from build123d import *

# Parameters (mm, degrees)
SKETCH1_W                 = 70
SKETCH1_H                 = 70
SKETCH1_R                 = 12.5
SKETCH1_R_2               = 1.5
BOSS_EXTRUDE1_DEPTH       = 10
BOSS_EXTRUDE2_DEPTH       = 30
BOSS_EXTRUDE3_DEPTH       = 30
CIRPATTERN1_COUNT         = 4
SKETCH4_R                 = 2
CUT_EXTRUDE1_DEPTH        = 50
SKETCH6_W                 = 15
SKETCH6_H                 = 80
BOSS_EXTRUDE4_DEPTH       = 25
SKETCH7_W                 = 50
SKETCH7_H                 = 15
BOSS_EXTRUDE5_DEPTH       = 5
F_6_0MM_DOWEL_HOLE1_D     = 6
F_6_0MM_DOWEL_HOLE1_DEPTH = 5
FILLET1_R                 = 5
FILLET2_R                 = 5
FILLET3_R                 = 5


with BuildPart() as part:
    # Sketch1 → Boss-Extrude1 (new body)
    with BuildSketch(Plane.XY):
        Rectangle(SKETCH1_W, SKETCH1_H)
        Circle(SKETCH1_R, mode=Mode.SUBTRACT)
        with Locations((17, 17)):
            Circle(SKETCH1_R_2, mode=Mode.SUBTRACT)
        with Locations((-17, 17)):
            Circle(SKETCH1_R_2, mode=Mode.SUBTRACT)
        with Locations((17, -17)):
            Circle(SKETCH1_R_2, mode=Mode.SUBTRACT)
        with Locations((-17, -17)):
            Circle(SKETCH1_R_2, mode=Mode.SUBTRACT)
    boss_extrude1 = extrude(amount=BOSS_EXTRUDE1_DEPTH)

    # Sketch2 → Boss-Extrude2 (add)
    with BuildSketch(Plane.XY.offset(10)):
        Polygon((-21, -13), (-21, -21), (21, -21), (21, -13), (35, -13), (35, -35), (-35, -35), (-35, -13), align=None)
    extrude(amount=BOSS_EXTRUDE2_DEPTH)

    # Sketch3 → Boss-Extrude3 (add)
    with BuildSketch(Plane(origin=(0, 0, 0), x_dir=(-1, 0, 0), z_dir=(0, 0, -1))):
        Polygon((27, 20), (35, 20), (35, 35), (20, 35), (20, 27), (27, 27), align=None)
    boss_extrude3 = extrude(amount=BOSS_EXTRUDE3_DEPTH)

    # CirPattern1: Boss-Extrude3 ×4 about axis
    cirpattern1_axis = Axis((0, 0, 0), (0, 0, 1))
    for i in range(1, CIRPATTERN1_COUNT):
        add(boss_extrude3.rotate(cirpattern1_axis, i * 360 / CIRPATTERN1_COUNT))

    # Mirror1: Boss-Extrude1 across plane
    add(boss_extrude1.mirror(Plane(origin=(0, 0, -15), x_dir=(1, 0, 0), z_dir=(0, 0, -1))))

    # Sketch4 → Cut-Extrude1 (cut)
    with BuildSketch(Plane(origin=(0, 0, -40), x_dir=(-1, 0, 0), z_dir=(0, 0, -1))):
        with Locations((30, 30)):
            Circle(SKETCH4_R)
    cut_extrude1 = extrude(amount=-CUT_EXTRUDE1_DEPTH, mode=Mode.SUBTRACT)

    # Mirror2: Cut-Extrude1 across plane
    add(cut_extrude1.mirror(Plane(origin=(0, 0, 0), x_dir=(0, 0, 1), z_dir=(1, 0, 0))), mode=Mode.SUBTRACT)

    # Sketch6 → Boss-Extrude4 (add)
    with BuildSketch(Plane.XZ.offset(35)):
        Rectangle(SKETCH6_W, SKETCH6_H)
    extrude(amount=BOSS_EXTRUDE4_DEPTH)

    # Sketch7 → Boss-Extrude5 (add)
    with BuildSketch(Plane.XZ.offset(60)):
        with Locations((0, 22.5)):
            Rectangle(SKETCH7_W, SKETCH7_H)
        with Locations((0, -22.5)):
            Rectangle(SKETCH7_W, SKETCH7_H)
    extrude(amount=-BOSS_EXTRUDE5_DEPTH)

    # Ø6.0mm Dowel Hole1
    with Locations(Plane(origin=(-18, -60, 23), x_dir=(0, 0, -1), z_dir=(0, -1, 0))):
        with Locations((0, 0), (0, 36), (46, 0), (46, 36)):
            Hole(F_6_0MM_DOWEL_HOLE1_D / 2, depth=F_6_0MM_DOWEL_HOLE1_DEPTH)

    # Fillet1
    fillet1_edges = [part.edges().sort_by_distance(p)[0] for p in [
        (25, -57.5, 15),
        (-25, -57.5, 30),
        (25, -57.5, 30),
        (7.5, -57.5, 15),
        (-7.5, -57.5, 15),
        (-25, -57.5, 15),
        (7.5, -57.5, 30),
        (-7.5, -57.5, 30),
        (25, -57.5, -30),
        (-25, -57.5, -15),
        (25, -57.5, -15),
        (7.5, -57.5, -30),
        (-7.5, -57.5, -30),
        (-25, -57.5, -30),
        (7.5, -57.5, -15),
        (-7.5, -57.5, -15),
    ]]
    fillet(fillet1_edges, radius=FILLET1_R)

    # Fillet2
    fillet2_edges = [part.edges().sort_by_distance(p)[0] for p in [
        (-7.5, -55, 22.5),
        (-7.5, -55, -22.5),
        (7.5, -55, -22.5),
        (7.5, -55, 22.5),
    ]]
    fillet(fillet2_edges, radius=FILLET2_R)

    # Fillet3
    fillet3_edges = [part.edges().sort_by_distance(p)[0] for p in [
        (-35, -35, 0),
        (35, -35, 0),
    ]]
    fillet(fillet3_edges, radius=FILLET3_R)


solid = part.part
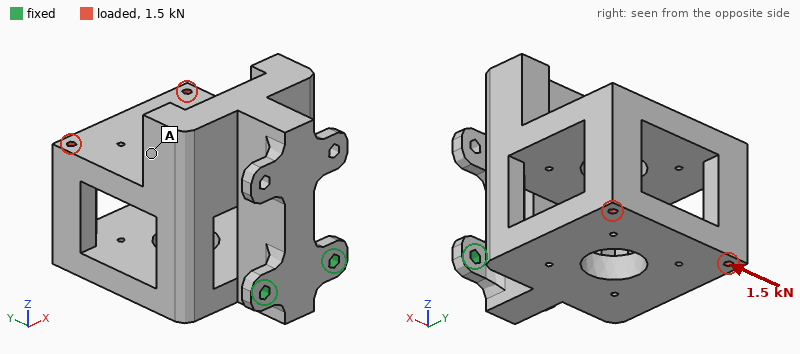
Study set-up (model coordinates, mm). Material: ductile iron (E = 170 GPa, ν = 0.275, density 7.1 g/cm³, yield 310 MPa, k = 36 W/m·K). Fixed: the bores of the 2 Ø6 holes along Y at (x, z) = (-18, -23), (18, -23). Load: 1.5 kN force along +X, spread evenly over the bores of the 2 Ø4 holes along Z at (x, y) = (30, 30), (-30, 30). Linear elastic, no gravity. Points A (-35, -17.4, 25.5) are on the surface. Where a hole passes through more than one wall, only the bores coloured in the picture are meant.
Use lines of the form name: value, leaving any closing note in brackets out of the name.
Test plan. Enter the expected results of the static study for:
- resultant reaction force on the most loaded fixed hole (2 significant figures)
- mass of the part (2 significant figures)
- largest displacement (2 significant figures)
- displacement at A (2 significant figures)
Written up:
resultant reaction force on the most loaded fixed hole: 5.0 kN
mass of the part: 1.3 kg
largest displacement: 0.35 mm
displacement at A: 0.18 mm
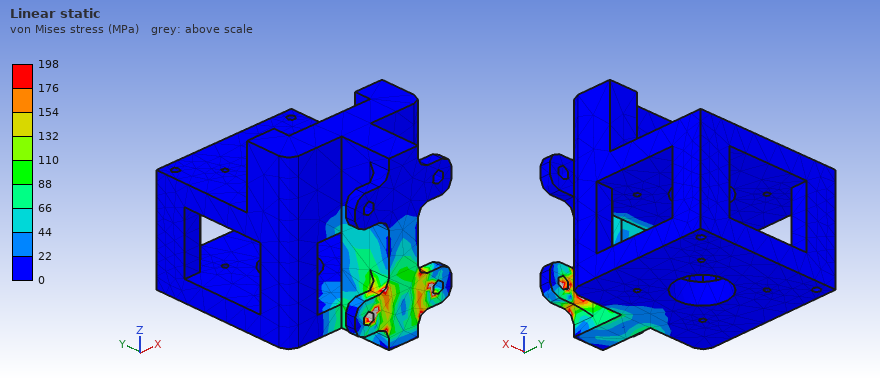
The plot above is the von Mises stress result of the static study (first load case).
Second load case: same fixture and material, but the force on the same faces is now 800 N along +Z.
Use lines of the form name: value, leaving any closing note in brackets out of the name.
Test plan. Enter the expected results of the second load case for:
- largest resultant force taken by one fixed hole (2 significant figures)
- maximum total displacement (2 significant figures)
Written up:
largest resultant force taken by one fixed hole: 410 N
maximum total displacement: 0.61 mm
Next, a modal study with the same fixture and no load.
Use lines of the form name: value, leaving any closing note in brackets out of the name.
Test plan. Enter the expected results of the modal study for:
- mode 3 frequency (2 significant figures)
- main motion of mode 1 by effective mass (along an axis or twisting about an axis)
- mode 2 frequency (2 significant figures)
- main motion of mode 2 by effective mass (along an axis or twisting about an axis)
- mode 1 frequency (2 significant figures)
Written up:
mode 3 frequency: 1100 Hz
main motion of mode 1 by effective mass: along Z
mode 2 frequency: 520 Hz
main motion of mode 2 by effective mass: along X
mode 1 frequency: 260 Hz
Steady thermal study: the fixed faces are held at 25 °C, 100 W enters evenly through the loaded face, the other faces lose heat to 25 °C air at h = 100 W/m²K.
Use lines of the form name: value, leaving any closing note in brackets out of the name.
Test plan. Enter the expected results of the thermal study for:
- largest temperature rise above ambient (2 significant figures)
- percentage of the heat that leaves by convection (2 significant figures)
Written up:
largest temperature rise above ambient: 80 K
percentage of the heat that leaves by convection: 98 %
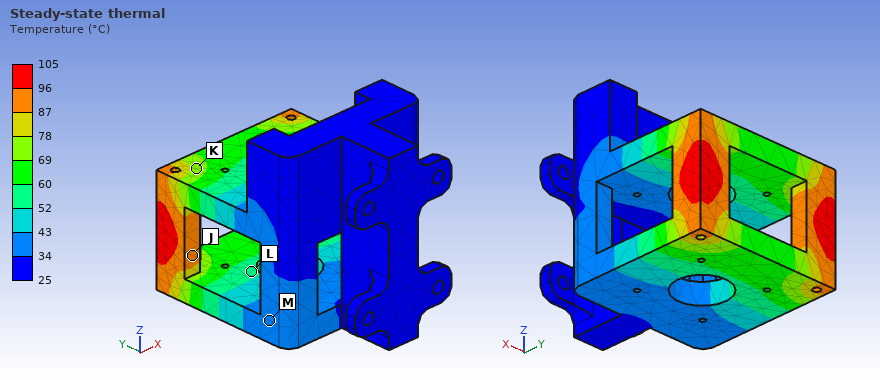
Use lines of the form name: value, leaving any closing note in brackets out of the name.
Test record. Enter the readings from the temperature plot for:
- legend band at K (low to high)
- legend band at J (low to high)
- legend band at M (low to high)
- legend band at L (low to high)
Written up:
legend band at K: 69 to 78 °C
legend band at J: 87 to 96 °C
legend band at M: 34 to 43 °C
legend band at L: 52 to 60 °C
